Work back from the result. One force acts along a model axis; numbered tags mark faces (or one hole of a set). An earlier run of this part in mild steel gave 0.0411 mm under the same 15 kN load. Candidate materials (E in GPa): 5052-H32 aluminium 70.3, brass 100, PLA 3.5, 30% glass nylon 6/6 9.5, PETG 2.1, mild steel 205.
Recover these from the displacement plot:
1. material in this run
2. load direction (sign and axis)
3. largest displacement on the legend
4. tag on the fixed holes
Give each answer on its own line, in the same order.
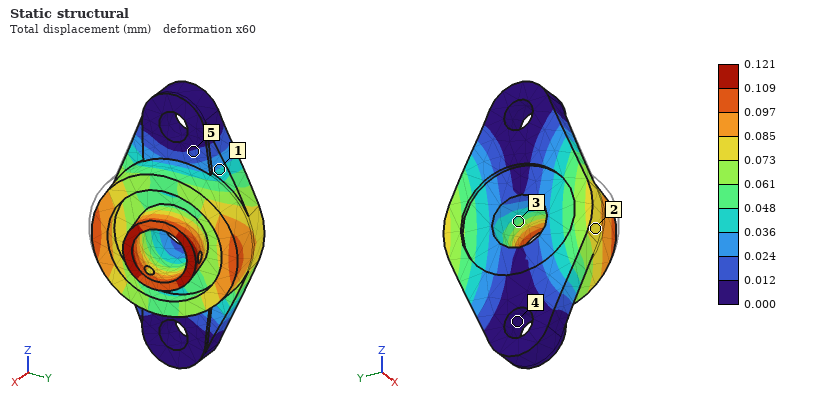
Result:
5052-H32 aluminium
+Y
0.121 mm
4
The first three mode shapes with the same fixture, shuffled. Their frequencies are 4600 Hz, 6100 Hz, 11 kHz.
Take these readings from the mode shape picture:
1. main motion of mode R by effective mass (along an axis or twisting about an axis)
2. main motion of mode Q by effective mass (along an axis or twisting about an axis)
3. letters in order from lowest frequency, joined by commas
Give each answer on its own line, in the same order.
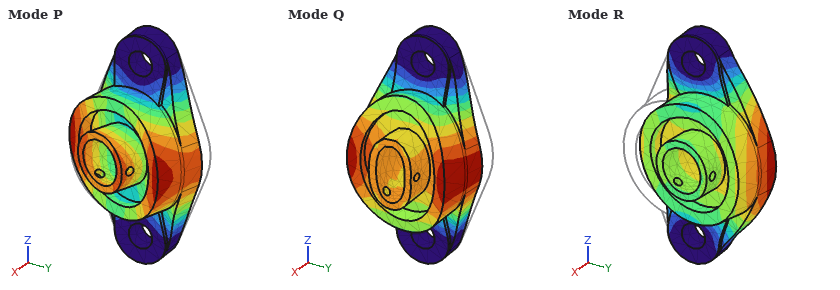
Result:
along Y
along X
P, Q, R
